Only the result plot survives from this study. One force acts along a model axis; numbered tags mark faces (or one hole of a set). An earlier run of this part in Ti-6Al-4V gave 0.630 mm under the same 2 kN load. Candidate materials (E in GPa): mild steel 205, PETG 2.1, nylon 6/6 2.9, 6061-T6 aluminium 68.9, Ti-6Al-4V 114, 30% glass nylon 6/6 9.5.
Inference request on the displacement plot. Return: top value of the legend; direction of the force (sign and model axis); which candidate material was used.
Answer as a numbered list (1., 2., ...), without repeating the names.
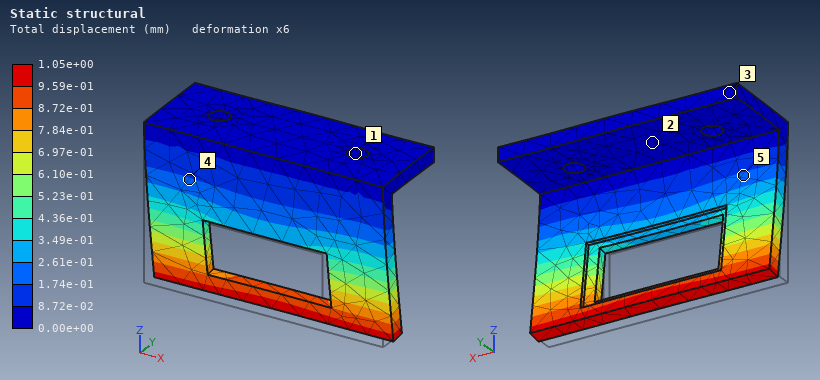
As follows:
1. 1.05e+00 mm
2. +Y
3. 6061-T6 aluminium
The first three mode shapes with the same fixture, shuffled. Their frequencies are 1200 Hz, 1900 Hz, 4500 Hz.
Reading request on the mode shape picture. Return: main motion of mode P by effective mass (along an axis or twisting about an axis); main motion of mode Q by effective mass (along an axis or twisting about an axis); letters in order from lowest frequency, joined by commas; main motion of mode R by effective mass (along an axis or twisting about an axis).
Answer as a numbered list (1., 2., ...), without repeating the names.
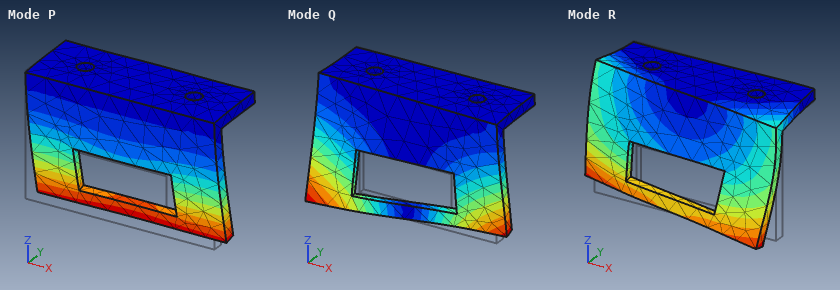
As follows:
1. along Y
2. twisting about Z
3. P, Q, R
4. along X
